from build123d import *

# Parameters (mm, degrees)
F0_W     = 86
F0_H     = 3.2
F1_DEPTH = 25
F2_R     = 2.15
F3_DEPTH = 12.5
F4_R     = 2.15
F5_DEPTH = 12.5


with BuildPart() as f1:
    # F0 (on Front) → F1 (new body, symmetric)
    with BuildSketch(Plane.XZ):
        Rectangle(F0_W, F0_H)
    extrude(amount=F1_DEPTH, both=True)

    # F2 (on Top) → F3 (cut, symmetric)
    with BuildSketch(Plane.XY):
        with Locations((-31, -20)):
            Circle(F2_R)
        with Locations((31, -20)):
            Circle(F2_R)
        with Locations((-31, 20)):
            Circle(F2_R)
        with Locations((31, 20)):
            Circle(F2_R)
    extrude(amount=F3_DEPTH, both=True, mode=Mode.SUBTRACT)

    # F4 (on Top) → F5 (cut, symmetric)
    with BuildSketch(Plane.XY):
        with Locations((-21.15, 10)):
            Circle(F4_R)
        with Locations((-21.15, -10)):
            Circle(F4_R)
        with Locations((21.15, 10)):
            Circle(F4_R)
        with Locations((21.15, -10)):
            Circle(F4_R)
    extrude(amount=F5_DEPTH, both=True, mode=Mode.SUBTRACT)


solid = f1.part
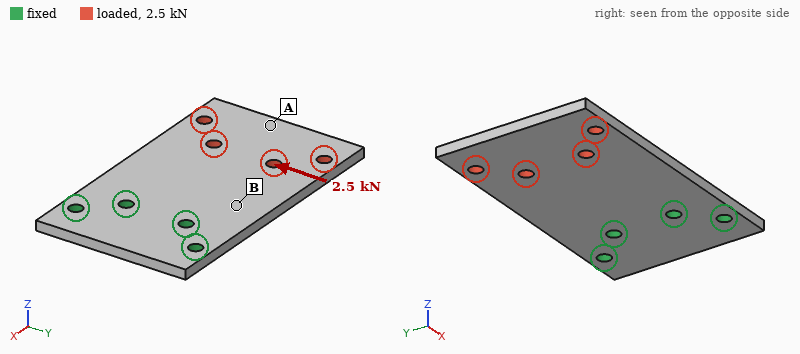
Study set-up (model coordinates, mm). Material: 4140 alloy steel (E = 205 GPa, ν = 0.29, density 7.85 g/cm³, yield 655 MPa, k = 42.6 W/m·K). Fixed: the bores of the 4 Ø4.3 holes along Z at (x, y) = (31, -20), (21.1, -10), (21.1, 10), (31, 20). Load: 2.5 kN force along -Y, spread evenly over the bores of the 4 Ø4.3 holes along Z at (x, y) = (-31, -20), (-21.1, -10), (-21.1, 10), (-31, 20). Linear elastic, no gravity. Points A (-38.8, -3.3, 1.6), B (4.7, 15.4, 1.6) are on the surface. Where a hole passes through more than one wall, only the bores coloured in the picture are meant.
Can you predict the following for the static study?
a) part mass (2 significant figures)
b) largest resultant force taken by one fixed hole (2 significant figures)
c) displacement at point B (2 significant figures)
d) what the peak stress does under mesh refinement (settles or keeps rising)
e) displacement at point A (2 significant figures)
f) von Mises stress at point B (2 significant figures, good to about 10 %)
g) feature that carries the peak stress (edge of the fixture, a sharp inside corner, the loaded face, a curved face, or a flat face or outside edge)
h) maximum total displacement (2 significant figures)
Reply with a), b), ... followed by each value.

a) 110 g
b) 2.3 kN
c) 9.5 µm
d) keeps rising
e) 36 µm
f) 43 MPa
g) edge of the fixture
h) 41 µm
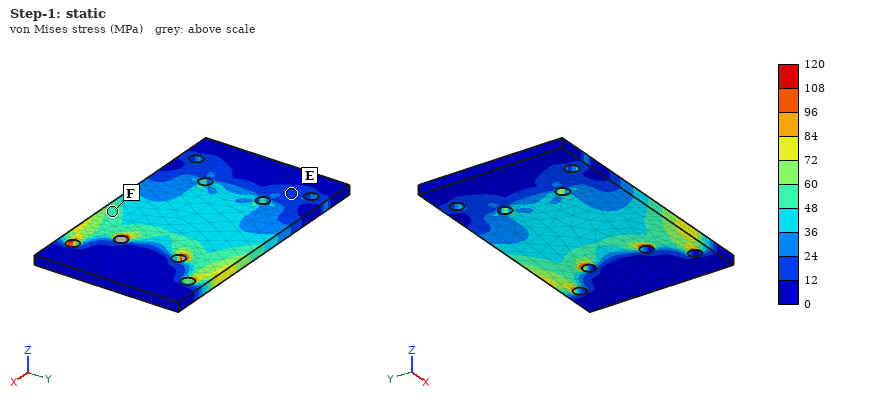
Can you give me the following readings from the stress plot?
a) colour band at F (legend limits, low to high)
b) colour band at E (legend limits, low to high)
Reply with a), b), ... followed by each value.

a) 48 to 60 MPa
b) 12 to 24 MPa
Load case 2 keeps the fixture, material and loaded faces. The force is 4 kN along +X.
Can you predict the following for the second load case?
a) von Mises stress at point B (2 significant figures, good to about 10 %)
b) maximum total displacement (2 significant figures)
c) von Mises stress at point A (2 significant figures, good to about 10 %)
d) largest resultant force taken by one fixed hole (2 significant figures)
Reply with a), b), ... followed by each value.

a) 26 MPa
b) 7.4 µm
c) 6.7 MPa
d) 1.4 kN
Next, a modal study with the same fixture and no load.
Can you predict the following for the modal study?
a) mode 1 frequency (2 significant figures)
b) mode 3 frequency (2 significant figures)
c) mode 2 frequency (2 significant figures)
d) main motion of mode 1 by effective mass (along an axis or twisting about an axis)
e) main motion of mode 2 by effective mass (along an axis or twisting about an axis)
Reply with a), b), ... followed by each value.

a) 670 Hz
b) 3900 Hz
c) 1800 Hz
d) along Z
e) twisting about X
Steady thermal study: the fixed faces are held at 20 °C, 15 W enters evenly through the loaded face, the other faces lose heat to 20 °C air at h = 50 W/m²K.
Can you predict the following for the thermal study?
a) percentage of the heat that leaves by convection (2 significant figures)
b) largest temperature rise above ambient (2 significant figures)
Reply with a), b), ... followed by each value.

a) 66 %
b) 54 K
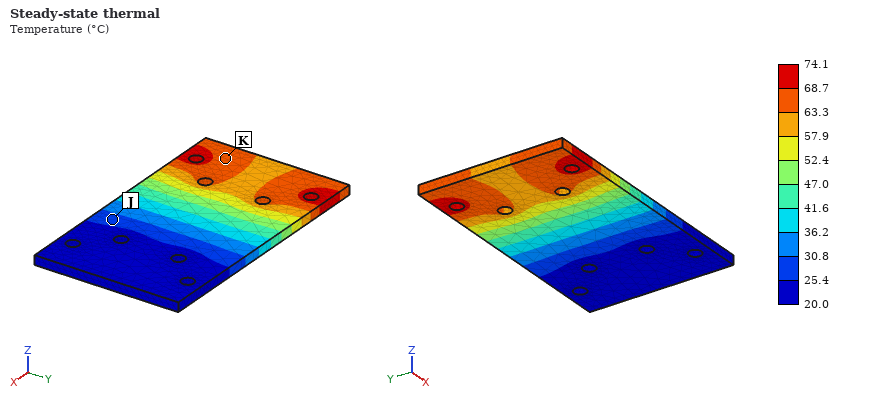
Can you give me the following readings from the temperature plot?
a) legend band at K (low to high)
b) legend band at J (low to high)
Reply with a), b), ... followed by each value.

a) 63.3 to 68.7 °C
b) 25.4 to 30.8 °C
